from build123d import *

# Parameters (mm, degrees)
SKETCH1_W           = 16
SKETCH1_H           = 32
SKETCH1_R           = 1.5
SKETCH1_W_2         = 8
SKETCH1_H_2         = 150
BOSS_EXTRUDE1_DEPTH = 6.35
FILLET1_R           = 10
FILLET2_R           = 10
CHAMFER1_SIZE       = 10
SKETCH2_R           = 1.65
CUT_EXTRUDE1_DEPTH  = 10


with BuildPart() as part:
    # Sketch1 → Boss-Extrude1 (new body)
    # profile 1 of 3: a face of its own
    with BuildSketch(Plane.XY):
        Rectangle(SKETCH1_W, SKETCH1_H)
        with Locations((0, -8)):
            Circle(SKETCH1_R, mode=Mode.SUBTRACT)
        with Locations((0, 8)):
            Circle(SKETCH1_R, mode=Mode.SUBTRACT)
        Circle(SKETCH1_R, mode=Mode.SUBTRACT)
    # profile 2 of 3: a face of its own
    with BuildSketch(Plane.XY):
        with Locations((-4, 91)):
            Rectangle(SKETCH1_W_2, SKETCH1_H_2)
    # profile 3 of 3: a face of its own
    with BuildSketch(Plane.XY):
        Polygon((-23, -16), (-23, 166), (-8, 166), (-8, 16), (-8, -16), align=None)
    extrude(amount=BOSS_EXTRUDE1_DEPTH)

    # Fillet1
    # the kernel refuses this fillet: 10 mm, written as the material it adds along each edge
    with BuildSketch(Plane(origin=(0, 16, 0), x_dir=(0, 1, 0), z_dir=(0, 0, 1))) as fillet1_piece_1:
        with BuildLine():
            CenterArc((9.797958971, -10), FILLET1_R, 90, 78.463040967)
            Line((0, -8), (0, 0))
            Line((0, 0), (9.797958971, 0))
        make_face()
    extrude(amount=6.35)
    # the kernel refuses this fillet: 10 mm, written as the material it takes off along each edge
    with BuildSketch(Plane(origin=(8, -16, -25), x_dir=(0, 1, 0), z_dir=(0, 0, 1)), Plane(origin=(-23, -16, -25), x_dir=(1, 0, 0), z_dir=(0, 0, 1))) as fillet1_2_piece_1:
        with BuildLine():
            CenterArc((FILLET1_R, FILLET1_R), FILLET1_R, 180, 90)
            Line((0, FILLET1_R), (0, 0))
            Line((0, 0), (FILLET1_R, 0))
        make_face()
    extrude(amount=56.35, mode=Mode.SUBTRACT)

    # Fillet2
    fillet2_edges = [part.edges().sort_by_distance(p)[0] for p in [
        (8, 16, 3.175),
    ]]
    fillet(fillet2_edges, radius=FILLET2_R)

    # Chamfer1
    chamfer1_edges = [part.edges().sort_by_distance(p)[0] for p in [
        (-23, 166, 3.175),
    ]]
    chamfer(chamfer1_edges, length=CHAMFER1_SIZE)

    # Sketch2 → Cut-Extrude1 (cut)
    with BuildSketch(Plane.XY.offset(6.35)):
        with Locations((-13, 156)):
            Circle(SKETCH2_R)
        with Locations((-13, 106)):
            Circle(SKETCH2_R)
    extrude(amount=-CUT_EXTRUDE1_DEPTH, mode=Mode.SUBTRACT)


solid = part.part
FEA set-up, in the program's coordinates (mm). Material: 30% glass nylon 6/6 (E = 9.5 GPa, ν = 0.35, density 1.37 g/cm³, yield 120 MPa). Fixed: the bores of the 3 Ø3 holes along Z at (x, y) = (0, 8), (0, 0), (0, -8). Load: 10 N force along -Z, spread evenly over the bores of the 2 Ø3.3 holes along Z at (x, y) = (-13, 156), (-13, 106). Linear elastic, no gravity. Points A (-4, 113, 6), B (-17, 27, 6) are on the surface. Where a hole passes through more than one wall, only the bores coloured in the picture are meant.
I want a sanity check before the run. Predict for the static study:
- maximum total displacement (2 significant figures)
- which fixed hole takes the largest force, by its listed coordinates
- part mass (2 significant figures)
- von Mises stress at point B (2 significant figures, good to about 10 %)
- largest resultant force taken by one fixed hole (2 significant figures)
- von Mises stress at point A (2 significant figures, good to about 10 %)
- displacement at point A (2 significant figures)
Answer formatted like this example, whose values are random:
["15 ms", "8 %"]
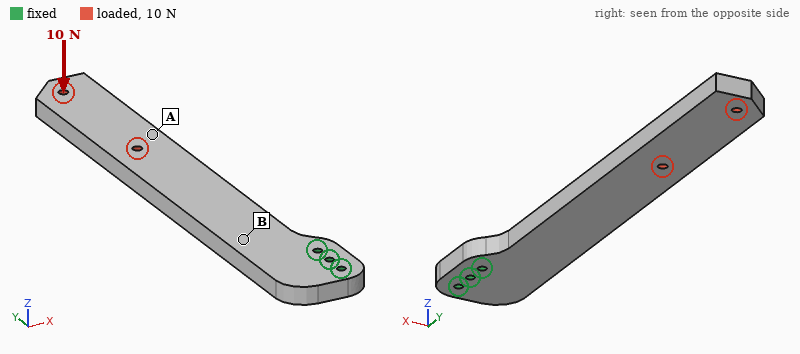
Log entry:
["2.0 mm", "(0, 8)", "38 g", "6.4 MPa", "64 N", "1.5 MPa", "1.1 mm"]
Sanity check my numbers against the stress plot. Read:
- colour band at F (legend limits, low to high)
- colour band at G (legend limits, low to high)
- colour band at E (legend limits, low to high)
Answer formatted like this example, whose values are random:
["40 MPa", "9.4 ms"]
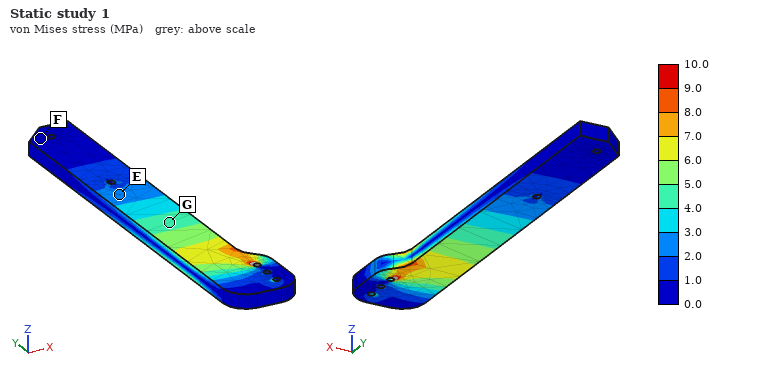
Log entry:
["0.0 to 1.0 MPa", "4.0 to 5.0 MPa", "2.0 to 3.0 MPa"]
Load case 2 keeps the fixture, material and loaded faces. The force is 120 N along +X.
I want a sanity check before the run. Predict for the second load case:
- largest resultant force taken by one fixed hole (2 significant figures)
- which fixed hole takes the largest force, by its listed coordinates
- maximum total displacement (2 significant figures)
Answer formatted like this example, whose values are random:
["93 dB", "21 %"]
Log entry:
["990 N", "(0, 8)", "2.0 mm"]
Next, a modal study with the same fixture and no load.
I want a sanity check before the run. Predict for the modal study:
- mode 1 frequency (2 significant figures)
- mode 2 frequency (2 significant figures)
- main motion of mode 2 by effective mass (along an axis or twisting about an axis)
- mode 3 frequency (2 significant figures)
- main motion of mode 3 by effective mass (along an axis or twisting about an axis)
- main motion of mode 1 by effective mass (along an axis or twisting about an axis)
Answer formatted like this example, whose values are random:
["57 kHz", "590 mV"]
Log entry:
["110 Hz", "370 Hz", "along X", "670 Hz", "along Z", "along Z"]
